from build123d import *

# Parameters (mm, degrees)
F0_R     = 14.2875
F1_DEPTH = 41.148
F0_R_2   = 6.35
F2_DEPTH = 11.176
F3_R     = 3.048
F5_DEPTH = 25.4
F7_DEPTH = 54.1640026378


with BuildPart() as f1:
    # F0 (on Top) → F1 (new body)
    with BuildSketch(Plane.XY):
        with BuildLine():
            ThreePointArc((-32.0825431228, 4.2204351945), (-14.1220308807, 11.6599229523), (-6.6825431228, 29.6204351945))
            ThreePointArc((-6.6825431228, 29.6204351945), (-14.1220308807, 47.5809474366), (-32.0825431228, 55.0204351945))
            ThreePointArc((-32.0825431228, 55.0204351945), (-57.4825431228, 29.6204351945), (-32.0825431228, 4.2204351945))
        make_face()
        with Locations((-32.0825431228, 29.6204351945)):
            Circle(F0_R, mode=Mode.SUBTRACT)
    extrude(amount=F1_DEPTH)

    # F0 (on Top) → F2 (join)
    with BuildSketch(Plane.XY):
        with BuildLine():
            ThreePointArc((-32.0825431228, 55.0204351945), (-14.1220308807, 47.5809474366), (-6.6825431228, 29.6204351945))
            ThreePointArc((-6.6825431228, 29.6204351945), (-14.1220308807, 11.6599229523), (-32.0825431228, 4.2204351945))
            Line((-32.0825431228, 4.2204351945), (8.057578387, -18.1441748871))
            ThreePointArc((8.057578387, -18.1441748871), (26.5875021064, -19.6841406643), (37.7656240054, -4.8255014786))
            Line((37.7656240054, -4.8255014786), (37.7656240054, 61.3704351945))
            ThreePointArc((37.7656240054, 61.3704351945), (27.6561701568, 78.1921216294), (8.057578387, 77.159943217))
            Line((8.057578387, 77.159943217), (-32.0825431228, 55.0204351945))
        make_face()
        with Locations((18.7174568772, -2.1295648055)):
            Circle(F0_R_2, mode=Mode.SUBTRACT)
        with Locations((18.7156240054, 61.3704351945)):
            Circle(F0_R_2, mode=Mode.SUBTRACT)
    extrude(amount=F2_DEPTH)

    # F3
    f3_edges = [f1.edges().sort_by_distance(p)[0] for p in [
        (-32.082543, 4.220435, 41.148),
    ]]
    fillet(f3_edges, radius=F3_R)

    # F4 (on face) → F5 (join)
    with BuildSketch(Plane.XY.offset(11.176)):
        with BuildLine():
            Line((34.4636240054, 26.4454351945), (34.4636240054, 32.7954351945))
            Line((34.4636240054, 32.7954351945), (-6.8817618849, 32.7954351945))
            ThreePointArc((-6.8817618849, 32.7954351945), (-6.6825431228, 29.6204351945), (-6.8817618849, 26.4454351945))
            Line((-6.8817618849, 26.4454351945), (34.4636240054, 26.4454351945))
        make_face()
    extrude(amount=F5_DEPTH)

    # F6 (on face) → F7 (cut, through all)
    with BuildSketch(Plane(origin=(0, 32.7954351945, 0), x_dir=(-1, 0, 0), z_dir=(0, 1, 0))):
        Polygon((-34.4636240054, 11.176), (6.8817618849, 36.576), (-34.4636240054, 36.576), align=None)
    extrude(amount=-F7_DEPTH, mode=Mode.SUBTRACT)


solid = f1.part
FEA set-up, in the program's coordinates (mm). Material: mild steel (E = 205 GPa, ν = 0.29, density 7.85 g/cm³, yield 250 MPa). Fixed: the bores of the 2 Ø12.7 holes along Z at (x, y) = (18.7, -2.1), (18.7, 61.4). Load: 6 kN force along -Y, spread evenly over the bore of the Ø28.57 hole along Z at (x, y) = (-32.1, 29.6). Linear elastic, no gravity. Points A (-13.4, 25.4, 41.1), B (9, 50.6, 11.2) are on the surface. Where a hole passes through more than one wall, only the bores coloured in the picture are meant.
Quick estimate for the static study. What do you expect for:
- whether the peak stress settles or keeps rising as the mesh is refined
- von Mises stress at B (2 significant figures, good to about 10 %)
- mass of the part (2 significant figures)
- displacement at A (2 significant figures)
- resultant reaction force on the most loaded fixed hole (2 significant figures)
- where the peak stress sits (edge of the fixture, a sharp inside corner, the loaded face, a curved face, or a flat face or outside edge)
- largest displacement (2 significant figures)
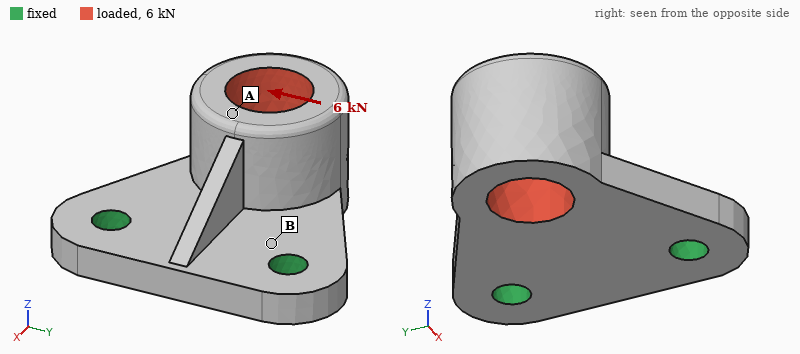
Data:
keeps rising
21 MPa
870 g
19 µm
5.5 kN
edge of the fixture
25 µm
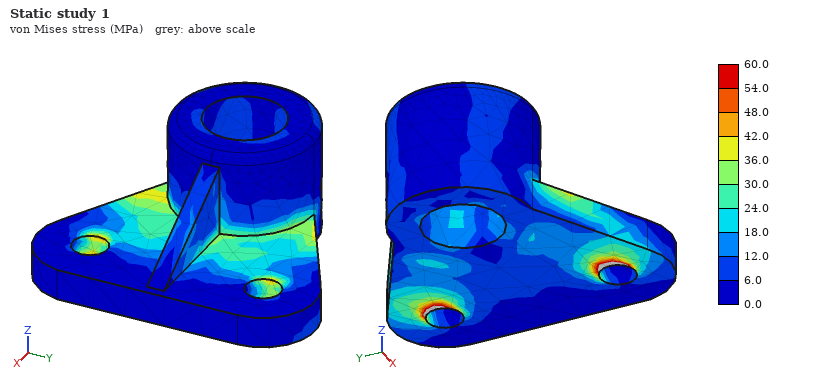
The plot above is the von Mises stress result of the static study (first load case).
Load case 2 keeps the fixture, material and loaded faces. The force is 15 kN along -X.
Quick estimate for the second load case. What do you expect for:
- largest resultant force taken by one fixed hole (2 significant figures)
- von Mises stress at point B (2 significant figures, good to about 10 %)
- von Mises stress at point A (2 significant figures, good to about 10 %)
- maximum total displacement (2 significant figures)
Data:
7.7 kN
97 MPa
34 MPa
0.15 mm
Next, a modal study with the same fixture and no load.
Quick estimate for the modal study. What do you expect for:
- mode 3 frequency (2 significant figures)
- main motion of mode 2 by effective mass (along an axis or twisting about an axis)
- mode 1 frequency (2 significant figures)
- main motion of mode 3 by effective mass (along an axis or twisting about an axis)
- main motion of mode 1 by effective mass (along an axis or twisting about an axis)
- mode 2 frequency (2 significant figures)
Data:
7000 Hz
along Y
1600 Hz
along Y
along Z
4000 Hz
